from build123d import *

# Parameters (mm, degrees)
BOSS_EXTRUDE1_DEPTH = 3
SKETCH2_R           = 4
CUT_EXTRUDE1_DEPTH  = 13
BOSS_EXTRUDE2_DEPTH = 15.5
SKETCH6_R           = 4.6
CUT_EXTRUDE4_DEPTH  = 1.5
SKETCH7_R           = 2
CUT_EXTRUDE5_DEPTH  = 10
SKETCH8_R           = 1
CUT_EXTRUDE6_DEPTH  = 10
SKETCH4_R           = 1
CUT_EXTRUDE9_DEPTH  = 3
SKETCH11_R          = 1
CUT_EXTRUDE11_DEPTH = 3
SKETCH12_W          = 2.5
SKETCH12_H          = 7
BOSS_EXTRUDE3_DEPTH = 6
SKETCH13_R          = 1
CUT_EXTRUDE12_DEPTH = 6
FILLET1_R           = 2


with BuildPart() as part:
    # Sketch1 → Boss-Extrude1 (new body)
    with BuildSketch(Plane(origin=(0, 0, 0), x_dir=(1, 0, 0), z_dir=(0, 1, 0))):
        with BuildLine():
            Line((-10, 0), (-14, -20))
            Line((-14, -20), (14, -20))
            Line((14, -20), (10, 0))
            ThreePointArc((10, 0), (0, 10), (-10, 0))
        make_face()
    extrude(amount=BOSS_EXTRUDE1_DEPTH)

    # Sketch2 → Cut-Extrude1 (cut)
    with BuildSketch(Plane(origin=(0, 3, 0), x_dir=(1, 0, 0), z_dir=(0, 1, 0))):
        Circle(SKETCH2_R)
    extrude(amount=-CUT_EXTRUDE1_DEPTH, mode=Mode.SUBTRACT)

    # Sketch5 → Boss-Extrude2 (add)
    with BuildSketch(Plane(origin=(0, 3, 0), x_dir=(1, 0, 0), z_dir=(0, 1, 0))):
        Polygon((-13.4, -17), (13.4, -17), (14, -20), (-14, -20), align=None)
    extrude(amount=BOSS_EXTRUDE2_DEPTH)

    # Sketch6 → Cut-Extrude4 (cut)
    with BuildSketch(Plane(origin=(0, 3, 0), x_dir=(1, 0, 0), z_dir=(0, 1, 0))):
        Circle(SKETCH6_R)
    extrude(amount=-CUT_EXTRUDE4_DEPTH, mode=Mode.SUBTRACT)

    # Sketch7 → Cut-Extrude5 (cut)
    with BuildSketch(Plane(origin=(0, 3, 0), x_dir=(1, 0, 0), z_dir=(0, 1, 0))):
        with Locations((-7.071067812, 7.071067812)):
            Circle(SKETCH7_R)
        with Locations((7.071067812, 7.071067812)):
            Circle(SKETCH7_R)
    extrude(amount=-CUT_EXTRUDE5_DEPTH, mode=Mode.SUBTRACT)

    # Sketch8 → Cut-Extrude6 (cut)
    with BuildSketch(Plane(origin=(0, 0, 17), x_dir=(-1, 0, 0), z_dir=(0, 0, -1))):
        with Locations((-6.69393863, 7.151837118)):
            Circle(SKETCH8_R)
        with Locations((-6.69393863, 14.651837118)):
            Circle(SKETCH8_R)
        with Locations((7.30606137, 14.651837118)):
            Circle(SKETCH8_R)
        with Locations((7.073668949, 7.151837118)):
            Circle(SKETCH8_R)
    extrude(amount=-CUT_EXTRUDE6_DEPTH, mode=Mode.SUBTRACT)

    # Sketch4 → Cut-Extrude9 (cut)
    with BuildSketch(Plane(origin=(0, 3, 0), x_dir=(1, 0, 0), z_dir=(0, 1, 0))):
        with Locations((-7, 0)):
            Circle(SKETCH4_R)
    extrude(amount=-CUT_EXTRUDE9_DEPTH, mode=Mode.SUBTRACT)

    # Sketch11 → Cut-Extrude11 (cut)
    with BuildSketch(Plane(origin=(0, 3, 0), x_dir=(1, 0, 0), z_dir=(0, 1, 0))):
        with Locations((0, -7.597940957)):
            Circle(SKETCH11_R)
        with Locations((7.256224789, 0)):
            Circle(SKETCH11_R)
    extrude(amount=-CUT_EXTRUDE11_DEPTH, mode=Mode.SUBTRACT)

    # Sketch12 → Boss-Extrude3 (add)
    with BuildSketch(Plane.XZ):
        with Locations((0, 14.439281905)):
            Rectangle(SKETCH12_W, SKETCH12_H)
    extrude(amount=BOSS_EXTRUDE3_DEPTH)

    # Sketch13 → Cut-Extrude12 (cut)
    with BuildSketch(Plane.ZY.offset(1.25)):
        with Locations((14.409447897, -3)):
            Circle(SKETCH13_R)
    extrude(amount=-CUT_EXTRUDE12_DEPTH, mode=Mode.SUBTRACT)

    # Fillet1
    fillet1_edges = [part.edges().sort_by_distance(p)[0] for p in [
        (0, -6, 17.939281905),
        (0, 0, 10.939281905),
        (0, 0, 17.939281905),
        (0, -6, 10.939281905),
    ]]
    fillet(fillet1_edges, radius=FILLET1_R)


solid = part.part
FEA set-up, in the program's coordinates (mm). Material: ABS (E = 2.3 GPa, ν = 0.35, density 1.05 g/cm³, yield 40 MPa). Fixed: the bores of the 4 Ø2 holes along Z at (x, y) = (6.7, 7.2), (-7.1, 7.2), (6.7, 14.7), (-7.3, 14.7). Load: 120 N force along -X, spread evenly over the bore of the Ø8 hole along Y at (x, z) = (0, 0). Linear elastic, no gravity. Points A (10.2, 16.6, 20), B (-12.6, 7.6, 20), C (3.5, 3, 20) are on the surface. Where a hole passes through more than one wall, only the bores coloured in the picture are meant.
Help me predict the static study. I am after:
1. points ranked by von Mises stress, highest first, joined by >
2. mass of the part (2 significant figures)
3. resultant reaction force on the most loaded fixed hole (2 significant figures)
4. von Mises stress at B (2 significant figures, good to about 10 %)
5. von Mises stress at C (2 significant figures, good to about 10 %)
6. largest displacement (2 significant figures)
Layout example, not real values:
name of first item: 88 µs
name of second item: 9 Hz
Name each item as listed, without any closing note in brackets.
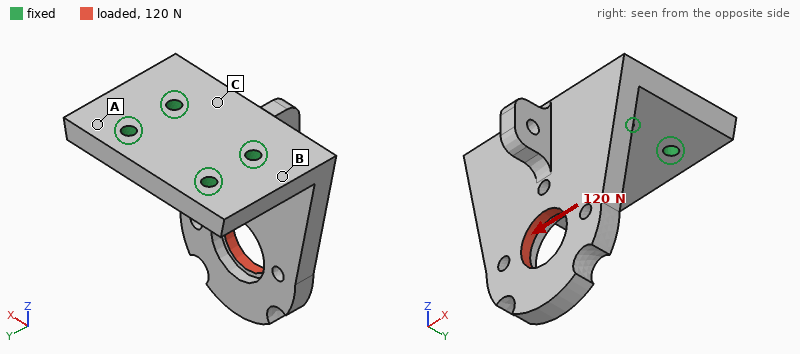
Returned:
points ranked by von Mises stress, highest first, joined by >: B > C > A
mass of the part: 3.2 g
resultant reaction force on the most loaded fixed hole: 160 N
von Mises stress at B: 12 MPa
von Mises stress at C: 8.6 MPa
largest displacement: 0.53 mm
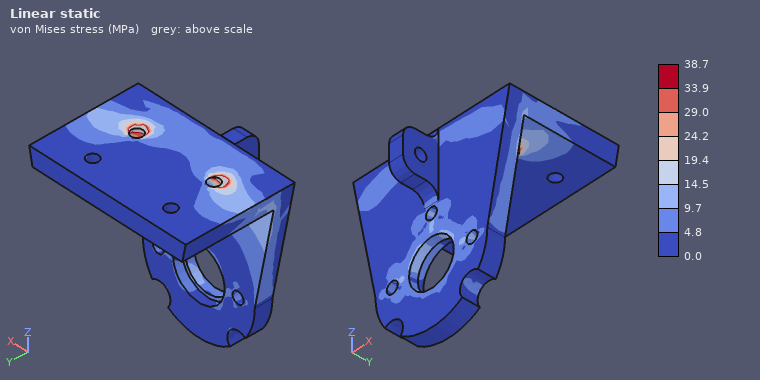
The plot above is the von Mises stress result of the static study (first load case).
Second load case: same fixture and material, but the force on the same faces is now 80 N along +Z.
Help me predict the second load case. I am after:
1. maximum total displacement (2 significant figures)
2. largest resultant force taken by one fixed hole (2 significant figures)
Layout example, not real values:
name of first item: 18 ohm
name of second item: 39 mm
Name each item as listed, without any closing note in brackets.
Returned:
maximum total displacement: 0.55 mm
largest resultant force taken by one fixed hole: 53 N
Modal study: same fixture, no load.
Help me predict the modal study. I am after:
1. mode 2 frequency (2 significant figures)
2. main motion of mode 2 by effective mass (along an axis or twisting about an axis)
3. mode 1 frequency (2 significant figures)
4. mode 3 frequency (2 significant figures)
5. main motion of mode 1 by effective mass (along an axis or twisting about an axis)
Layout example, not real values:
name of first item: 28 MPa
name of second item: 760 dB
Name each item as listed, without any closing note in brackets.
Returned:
mode 2 frequency: 2600 Hz
main motion of mode 2 by effective mass: along X
mode 1 frequency: 1000 Hz
mode 3 frequency: 3600 Hz
main motion of mode 1 by effective mass: along Y
